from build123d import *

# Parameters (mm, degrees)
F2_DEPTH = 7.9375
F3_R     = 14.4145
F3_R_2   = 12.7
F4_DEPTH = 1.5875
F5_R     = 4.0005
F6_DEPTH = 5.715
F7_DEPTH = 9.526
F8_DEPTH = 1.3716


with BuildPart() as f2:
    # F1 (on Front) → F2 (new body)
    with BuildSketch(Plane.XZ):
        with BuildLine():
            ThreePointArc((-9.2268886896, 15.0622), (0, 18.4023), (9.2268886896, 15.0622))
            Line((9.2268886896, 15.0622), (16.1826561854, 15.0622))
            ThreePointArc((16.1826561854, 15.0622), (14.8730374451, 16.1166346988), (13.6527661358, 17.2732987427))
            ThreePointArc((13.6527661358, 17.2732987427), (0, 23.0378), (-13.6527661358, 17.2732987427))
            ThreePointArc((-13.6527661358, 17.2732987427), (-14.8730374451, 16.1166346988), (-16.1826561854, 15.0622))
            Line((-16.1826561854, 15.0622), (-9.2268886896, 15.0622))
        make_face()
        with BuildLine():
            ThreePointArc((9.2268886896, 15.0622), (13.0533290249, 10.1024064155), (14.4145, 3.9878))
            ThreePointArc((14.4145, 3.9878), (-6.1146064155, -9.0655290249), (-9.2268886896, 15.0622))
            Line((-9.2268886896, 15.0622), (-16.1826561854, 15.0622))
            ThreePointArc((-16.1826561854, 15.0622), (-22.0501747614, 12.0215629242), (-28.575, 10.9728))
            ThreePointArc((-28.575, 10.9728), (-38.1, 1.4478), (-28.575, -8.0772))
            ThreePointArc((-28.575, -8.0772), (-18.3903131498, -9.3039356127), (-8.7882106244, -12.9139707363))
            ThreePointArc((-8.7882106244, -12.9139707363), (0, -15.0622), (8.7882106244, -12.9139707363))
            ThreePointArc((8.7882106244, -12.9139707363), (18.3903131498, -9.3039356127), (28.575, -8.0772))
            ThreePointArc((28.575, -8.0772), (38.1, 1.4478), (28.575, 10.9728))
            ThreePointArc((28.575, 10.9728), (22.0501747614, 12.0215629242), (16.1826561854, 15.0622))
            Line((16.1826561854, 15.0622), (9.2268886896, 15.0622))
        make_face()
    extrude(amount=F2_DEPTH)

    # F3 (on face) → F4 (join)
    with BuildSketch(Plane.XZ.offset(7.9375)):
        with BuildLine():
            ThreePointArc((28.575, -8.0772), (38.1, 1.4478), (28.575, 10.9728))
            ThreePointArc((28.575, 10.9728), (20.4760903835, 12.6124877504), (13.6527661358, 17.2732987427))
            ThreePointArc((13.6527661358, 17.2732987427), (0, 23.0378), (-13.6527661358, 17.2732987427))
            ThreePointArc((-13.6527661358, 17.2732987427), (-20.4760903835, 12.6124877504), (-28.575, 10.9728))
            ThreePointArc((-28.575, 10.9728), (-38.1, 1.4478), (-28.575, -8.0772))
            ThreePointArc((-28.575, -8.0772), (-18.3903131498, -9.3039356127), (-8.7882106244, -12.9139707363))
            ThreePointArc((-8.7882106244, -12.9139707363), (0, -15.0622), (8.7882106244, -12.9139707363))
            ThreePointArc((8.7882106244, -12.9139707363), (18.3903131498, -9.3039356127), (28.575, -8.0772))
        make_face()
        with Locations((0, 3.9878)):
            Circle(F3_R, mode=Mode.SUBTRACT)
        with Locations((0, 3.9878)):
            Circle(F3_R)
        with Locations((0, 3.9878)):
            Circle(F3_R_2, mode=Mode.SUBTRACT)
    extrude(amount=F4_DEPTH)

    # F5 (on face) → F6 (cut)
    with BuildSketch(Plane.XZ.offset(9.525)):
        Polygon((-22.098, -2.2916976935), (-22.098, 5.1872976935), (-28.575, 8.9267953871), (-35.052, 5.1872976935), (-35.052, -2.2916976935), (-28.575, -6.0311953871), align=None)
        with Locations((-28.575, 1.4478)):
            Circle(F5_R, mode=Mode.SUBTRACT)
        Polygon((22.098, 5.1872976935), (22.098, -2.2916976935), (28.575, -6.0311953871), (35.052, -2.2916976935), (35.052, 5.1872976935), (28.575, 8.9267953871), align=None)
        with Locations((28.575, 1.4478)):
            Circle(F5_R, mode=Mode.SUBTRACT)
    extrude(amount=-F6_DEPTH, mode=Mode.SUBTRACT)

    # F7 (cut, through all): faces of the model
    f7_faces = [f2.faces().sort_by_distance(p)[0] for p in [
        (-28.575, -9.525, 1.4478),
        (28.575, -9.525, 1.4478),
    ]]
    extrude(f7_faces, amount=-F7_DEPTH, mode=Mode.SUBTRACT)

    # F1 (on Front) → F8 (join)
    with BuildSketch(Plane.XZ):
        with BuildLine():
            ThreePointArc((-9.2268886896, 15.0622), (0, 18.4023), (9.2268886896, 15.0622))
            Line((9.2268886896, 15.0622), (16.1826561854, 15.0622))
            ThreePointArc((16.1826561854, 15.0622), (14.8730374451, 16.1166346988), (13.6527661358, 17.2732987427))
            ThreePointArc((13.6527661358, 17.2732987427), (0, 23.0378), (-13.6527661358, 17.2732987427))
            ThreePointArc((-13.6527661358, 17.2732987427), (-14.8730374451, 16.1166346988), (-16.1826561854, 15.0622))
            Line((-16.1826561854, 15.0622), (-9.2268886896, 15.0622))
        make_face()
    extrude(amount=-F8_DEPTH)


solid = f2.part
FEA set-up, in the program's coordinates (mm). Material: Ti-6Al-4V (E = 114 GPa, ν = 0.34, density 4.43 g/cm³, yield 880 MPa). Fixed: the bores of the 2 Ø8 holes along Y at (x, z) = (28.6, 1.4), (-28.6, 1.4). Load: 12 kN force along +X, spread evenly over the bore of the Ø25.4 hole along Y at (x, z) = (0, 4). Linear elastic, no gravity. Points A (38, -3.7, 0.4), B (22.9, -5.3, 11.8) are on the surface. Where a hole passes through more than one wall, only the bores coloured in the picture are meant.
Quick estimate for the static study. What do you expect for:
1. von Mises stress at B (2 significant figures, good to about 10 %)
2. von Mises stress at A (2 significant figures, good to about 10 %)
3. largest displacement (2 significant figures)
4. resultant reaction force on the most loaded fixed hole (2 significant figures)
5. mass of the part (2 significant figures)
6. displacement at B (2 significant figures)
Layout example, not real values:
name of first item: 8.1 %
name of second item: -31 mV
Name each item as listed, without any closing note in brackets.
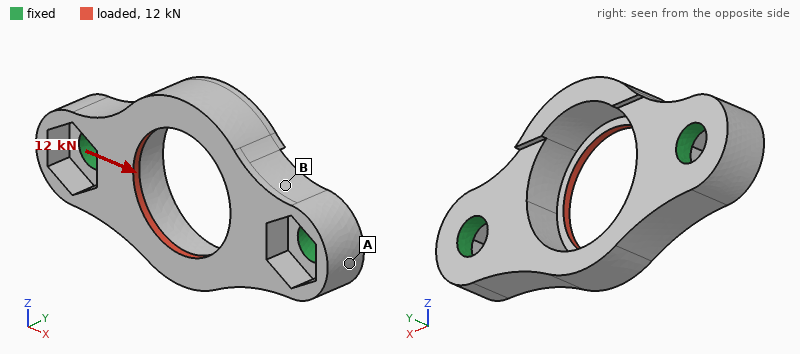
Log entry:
von Mises stress at B: 94 MPa
von Mises stress at A: 23 MPa
largest displacement: 36 µm
resultant reaction force on the most loaded fixed hole: 6.1 kN
mass of the part: 45 g
displacement at B: 11 µm
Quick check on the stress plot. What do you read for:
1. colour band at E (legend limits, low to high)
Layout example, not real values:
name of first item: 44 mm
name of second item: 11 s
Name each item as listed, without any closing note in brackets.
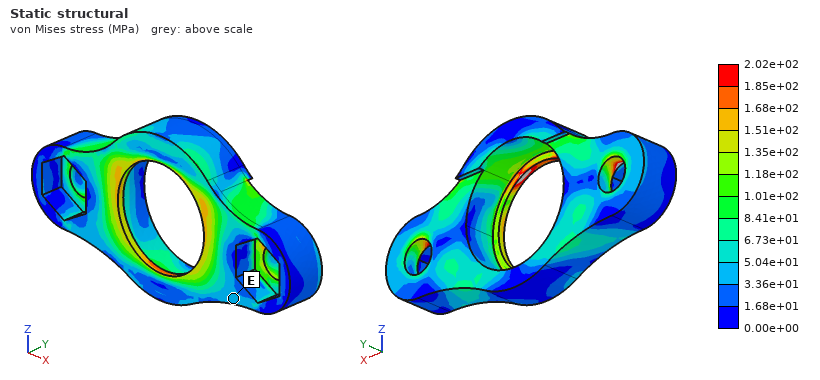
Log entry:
colour band at E: 3.36e+01 to 5.04e+01 MPa
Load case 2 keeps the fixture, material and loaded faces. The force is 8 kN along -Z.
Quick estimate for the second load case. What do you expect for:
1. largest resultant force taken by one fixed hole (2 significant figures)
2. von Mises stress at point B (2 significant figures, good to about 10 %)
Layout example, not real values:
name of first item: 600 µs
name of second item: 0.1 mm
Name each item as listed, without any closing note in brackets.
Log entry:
largest resultant force taken by one fixed hole: 4.0 kN
von Mises stress at point B: 70 MPa
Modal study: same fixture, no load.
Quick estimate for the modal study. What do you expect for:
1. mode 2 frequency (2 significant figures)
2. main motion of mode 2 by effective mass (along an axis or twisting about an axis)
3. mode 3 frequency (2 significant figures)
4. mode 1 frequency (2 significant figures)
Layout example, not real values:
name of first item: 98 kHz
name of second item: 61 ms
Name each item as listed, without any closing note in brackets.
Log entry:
mode 2 frequency: 9800 Hz
main motion of mode 2 by effective mass: along Y
mode 3 frequency: 18 kHz
mode 1 frequency: 7400 Hz
